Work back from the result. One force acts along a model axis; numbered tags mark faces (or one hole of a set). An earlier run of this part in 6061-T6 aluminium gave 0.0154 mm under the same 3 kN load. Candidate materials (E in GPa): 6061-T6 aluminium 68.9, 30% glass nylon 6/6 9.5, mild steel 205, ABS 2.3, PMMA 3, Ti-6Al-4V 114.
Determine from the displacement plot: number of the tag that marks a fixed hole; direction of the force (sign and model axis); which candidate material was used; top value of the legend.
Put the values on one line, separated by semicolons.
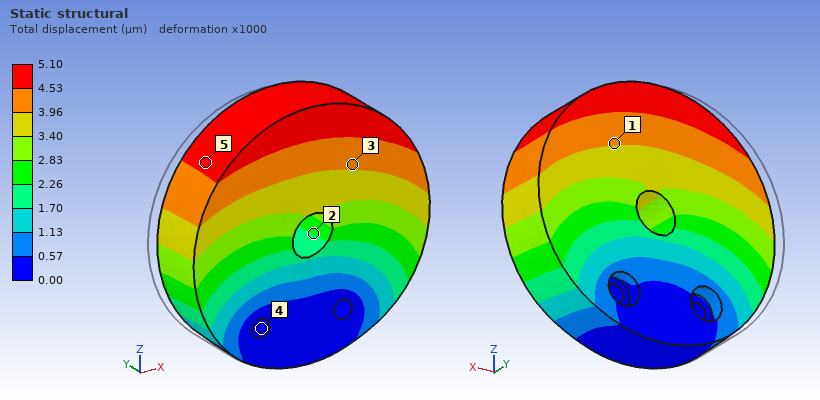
4; +X; mild steel; 5.10 µm
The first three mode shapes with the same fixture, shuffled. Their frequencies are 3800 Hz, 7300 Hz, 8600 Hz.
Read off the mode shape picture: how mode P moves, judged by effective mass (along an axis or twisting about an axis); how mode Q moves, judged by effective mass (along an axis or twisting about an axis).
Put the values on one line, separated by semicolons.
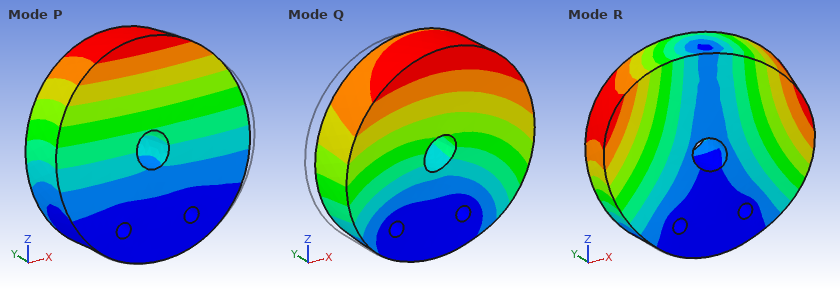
along Y; along X
